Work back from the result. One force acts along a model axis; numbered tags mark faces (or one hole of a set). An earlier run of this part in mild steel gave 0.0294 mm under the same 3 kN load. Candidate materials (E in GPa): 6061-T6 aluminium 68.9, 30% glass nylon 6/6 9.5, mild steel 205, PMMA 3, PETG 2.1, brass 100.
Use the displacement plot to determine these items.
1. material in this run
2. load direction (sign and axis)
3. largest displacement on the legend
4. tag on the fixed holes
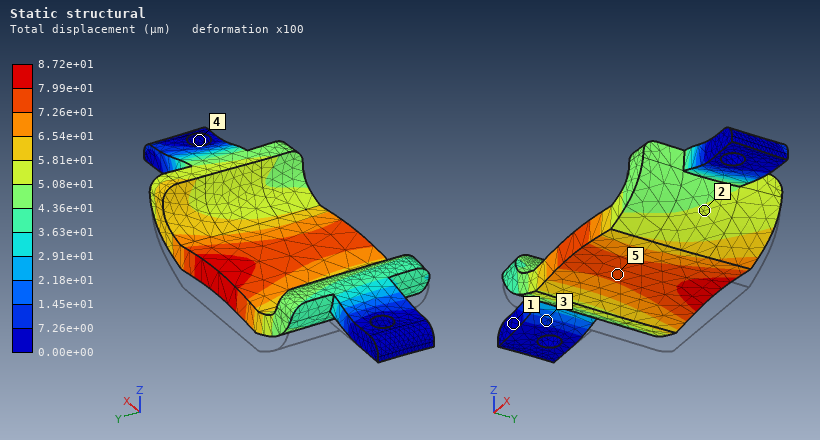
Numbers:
6061-T6 aluminium
+Z
8.72e+01 µm
4
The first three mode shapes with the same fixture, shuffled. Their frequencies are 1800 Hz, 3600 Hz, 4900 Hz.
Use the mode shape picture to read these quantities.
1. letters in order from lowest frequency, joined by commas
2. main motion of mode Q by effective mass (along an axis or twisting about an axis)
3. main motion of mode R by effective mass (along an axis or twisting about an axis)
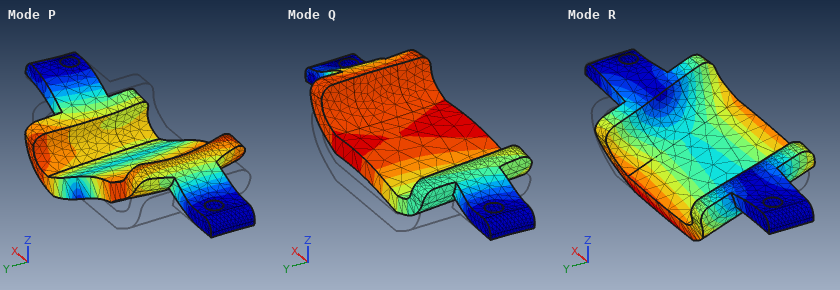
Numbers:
R, Q, P
along Z
along Y
